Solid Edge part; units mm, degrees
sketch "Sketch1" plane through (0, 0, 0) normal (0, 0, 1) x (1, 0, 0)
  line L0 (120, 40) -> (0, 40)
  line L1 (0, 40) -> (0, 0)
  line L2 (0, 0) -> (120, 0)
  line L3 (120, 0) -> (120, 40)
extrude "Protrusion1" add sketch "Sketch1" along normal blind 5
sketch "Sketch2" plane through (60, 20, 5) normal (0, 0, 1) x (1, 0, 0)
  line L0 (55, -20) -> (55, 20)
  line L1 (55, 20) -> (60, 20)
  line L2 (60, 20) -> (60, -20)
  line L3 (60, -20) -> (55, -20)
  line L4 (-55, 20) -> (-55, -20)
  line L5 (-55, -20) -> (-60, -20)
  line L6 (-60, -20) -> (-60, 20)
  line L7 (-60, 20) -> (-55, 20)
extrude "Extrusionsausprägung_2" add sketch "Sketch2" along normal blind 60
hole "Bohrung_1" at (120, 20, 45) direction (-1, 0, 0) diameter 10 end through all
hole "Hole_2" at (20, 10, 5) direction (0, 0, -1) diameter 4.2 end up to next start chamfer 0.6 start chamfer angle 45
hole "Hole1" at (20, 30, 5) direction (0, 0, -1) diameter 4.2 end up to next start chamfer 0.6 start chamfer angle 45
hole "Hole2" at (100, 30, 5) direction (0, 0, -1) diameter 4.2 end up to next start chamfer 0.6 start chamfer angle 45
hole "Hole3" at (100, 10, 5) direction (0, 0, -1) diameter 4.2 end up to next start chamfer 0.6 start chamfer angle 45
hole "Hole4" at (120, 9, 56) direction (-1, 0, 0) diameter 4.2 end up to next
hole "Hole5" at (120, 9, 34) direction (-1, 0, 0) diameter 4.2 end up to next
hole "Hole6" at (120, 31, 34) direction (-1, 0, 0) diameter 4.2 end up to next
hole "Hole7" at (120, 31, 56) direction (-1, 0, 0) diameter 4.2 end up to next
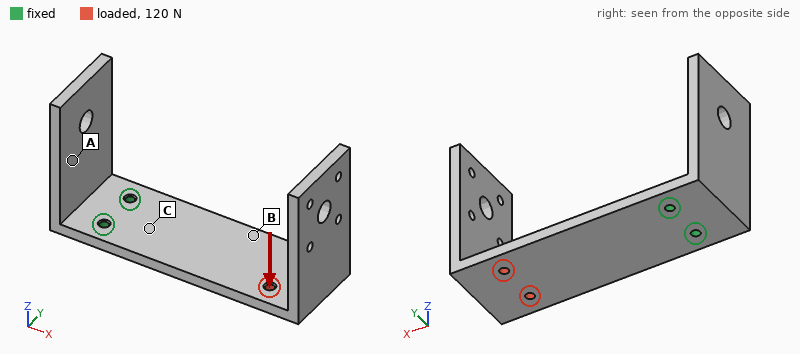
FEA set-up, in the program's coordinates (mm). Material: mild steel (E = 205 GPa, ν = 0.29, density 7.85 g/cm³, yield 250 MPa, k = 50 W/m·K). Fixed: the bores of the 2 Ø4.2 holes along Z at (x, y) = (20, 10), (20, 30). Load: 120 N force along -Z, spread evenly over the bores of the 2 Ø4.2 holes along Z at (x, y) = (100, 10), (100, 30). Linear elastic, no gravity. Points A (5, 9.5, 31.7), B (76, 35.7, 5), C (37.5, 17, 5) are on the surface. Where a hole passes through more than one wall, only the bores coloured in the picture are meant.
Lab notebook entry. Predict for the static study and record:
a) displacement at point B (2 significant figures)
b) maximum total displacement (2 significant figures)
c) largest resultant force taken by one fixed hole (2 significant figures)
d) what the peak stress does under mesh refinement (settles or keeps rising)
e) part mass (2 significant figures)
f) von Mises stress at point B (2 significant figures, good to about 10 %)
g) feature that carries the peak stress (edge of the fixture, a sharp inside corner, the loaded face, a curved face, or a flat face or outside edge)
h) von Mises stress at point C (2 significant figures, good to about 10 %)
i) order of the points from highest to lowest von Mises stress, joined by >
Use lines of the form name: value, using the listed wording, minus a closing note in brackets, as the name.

displacement at point B: 0.14 mm
maximum total displacement: 0.43 mm
largest resultant force taken by one fixed hole: 61 N
what the peak stress does under mesh refinement: keeps rising
part mass: 370 g
von Mises stress at point B: 17 MPa
feature that carries the peak stress: edge of the fixture
von Mises stress at point C: 42 MPa
order of the points from highest to lowest von Mises stress, joined by >: C > B > A
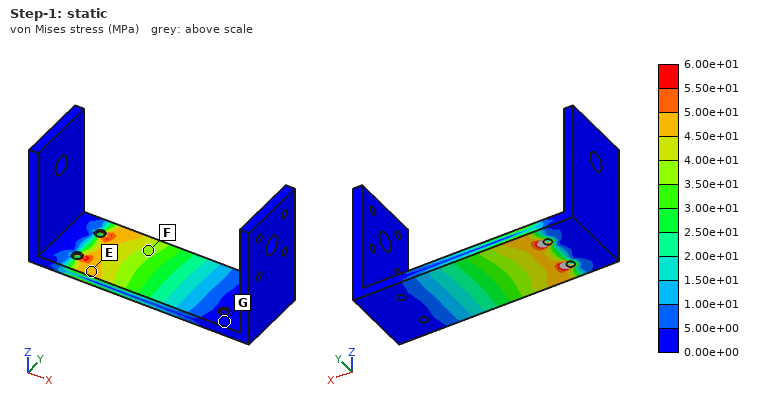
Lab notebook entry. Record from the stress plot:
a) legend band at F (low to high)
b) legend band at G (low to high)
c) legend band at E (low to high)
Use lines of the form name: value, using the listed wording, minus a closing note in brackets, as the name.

legend band at F: 3.50e+01 to 4.00e+01 MPa
legend band at G: 0.00e+00 to 5.00e+00 MPa
legend band at E: 4.50e+01 to 5.00e+01 MPa
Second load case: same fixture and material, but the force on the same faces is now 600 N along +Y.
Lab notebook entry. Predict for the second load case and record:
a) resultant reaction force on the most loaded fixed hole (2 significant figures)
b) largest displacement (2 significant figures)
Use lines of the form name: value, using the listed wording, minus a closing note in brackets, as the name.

resultant reaction force on the most loaded fixed hole: 2.2 kN
largest displacement: 37 µm
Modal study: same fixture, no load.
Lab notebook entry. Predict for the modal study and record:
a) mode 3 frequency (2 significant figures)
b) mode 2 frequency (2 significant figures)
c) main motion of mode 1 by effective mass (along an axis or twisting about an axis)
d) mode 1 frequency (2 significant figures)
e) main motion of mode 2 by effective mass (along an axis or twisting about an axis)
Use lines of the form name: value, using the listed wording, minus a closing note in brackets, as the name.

mode 3 frequency: 720 Hz
mode 2 frequency: 500 Hz
main motion of mode 1 by effective mass: along Z
mode 1 frequency: 210 Hz
main motion of mode 2 by effective mass: along Y
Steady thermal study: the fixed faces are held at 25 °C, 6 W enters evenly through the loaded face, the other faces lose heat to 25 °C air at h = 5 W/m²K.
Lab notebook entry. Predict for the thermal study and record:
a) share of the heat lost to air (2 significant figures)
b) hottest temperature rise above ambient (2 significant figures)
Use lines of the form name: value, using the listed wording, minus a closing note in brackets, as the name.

share of the heat lost to air: 31 %
hottest temperature rise above ambient: 37 K
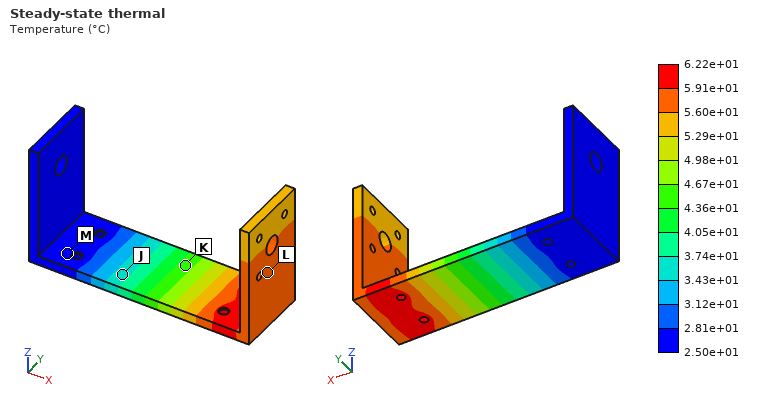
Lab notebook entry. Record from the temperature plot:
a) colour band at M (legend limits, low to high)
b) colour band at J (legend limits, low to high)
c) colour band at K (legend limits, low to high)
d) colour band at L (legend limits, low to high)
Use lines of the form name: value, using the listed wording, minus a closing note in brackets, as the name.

colour band at M: 2.50e+01 to 2.81e+01 °C
colour band at J: 3.43e+01 to 3.74e+01 °C
colour band at K: 4.36e+01 to 4.67e+01 °C
colour band at L: 5.60e+01 to 5.91e+01 °C
